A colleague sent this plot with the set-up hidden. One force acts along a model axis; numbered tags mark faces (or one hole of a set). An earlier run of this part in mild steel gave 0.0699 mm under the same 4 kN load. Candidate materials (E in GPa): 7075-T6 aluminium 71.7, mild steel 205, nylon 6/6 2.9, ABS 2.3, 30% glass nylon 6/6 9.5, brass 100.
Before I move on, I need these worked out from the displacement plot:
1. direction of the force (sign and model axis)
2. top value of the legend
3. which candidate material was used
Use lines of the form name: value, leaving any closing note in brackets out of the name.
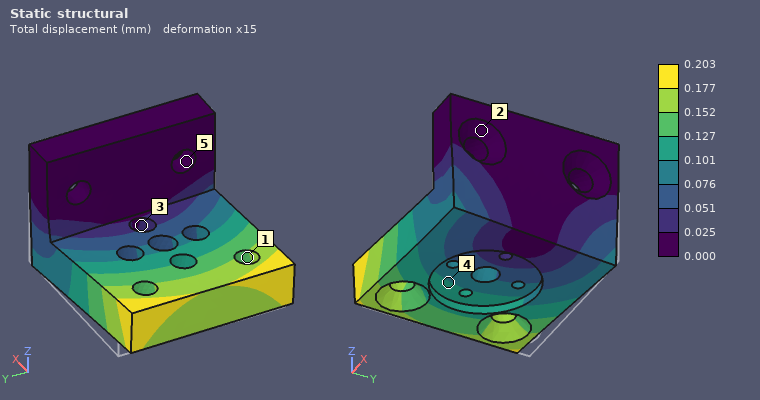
direction of the force: -Y
top value of the legend: 0.203 mm
which candidate material was used: 7075-T6 aluminium
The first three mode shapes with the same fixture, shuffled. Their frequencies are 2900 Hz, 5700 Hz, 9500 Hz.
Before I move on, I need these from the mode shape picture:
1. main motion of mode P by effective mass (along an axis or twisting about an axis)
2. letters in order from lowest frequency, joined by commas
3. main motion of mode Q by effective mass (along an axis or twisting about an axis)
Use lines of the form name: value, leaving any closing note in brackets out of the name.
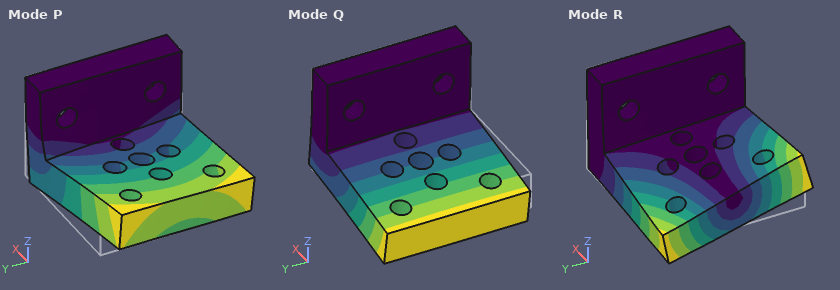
main motion of mode P by effective mass: along Y
letters in order from lowest frequency, joined by commas: Q, P, R
main motion of mode Q by effective mass: along Z
